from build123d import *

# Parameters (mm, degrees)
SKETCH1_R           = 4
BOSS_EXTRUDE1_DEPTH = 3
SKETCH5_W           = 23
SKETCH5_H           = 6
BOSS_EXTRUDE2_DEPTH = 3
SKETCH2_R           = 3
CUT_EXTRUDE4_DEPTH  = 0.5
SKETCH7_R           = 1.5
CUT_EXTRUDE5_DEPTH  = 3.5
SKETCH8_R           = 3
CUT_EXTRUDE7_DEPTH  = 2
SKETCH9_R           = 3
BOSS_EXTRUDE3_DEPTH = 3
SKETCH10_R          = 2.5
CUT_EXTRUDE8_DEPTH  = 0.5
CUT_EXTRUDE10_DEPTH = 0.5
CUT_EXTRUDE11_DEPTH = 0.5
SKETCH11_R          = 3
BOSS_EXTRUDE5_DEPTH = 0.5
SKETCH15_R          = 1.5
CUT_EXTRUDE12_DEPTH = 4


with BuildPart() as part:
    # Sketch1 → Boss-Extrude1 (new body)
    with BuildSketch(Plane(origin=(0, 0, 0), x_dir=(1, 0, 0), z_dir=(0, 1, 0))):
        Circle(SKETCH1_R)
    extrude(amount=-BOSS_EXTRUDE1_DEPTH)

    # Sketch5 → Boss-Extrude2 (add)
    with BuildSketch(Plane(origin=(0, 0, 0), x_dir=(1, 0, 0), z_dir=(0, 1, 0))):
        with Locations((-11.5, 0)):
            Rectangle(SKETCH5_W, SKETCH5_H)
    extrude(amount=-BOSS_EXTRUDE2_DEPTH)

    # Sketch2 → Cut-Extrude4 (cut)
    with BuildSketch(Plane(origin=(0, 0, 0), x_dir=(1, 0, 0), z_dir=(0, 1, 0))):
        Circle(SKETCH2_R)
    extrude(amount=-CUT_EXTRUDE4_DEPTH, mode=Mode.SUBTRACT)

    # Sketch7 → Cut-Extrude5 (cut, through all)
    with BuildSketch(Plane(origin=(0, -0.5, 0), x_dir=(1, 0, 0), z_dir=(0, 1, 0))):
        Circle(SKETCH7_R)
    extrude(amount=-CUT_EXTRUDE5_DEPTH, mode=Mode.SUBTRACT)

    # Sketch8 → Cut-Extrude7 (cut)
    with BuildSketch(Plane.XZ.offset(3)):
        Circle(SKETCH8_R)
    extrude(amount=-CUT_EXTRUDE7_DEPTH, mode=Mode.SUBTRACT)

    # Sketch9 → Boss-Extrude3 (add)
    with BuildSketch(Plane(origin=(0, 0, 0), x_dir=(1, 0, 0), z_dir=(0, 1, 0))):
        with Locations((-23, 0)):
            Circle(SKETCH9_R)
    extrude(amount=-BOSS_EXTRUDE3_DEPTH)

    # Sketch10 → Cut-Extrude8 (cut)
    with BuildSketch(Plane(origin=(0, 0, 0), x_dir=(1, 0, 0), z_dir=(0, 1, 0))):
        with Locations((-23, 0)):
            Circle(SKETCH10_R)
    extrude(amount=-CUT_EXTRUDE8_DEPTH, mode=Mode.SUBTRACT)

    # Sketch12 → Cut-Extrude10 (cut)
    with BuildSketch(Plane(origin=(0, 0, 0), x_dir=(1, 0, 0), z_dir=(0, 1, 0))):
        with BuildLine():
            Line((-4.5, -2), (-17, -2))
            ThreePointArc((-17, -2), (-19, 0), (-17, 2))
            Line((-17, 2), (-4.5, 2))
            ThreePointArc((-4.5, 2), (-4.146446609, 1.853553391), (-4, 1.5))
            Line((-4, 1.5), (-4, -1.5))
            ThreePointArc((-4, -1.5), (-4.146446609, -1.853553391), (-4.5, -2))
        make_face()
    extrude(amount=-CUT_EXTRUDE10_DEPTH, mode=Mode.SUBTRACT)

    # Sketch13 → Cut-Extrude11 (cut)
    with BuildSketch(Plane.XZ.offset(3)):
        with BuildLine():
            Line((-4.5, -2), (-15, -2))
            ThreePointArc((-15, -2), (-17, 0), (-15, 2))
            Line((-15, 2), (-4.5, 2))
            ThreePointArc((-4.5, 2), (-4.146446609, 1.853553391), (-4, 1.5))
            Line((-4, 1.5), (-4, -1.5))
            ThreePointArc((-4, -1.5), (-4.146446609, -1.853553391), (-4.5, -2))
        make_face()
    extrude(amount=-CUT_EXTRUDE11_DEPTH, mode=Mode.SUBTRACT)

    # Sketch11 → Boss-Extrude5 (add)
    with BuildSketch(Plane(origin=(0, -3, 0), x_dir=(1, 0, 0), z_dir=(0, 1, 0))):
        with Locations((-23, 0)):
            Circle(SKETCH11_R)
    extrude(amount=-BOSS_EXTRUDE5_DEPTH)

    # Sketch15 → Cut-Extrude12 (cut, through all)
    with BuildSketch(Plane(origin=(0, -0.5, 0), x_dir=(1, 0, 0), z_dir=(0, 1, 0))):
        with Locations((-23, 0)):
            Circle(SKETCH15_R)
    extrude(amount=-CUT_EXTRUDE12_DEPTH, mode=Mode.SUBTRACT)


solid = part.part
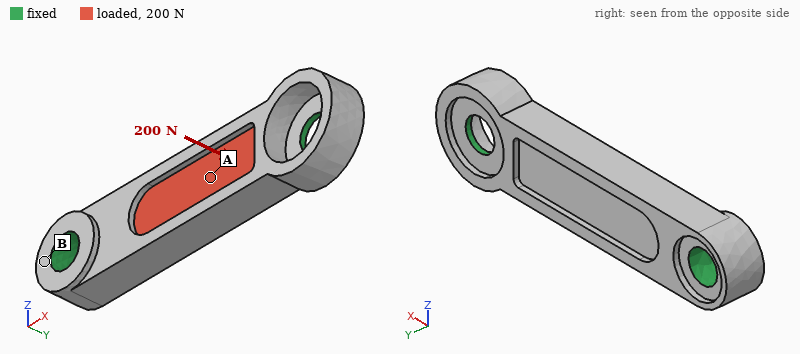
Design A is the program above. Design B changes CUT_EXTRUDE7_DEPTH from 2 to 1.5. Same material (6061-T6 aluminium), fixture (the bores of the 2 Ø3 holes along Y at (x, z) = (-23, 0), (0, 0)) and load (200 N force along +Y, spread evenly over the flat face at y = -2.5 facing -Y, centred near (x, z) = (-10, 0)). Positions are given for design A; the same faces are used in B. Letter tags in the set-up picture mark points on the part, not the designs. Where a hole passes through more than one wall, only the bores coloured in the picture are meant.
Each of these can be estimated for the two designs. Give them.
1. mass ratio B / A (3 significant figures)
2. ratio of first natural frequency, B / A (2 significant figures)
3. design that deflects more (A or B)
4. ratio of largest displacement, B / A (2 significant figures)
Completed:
1.03
1.2
A
0.79
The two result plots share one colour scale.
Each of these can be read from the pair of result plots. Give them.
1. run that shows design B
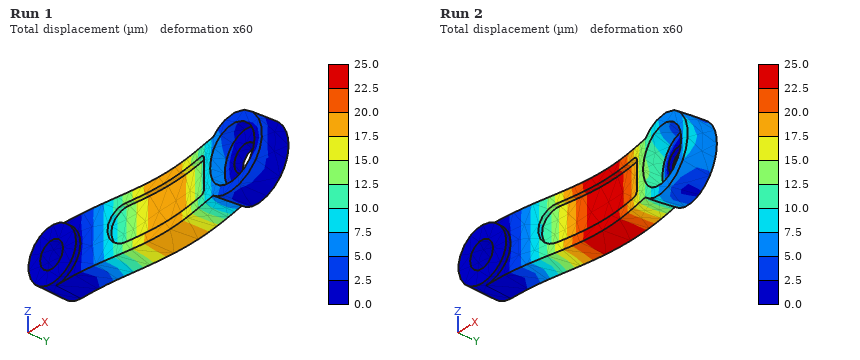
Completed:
Run 1
